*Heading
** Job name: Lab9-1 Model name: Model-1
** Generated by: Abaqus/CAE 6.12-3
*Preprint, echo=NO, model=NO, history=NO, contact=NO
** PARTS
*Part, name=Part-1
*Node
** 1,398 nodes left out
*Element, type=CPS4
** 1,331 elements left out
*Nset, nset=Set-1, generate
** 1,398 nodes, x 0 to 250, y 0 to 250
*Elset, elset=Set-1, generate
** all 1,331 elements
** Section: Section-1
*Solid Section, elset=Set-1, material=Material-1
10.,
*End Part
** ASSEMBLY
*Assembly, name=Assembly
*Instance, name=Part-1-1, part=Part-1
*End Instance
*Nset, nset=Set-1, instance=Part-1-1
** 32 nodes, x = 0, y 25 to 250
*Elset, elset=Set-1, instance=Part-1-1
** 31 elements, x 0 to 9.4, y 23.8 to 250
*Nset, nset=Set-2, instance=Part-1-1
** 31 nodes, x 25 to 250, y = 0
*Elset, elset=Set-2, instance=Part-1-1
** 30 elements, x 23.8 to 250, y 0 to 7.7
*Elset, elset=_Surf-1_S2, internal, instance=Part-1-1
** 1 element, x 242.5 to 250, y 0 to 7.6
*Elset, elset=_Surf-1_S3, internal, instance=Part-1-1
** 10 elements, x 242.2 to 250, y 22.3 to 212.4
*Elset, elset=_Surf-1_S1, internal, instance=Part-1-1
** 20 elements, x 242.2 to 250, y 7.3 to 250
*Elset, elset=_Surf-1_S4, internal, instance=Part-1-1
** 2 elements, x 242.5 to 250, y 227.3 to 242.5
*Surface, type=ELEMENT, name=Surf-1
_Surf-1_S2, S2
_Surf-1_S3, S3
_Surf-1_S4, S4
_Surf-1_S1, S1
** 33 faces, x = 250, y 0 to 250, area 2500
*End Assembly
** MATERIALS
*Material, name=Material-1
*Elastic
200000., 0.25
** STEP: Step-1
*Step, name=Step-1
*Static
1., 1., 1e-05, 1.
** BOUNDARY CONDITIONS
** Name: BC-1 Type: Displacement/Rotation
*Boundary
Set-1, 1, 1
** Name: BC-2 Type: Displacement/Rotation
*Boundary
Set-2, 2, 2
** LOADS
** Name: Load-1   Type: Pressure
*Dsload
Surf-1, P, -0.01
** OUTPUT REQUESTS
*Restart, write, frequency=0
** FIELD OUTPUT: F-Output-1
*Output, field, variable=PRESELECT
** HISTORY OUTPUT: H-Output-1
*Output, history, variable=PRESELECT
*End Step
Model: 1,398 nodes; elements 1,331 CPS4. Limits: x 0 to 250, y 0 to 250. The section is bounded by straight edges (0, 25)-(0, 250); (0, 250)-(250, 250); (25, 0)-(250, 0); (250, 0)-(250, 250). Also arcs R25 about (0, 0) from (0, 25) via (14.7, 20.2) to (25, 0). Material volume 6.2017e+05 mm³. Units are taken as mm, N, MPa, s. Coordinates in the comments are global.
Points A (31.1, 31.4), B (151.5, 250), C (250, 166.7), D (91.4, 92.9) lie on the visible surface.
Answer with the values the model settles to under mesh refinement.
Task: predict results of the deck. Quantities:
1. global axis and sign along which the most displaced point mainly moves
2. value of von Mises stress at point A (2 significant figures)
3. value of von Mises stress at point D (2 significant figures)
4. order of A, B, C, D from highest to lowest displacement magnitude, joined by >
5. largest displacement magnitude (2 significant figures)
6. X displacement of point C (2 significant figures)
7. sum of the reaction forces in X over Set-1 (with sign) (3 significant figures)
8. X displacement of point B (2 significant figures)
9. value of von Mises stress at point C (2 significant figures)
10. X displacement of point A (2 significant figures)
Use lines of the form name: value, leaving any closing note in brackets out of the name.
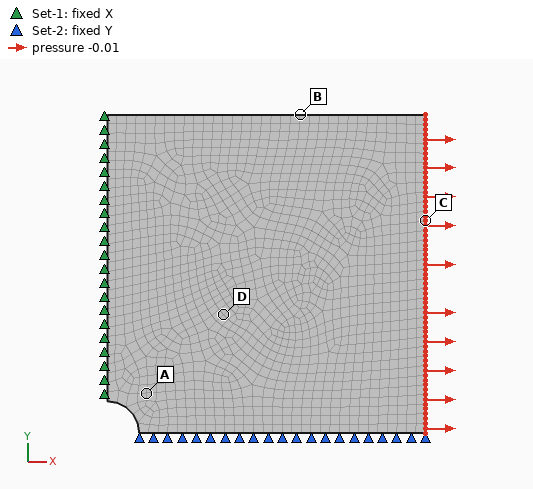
global axis and sign along which the most displaced point mainly moves: +X
value of von Mises stress at point A: 0.013 MPa
value of von Mises stress at point D: 0.011 MPa
order of A, B, C, D from highest to lowest displacement magnitude, joined by >: C > B > D > A
largest displacement magnitude: 1.3e-05 mm
X displacement of point C: 1.3e-05 mm
sum of the reaction forces in X over Set-1 (with sign): -25.0 N
X displacement of point B: 7.4e-06 mm
value of von Mises stress at point C: 0.010 MPa
X displacement of point A: 2.4e-06 mm
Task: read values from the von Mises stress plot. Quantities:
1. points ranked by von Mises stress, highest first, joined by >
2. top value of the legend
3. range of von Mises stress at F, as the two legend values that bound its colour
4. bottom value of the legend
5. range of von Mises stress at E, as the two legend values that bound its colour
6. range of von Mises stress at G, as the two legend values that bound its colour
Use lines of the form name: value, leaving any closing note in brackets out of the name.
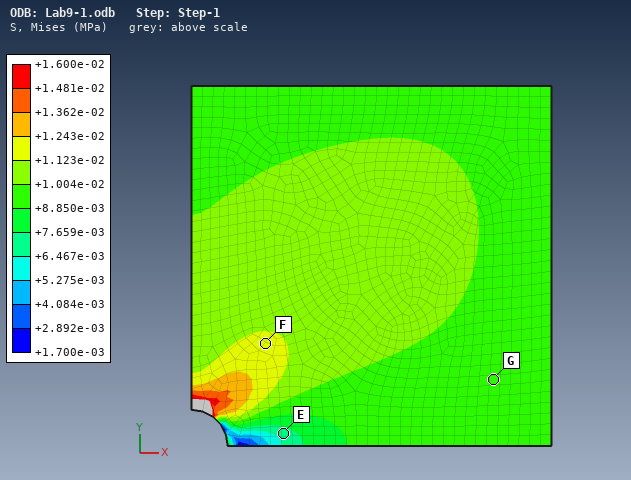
points ranked by von Mises stress, highest first, joined by >: F > G > E
top value of the legend: +1.600e-02 MPa
range of von Mises stress at F, as the two legend values that bound its colour: +1.123e-02 to +1.243e-02 MPa
bottom value of the legend: +1.700e-03 MPa
range of von Mises stress at E, as the two legend values that bound its colour: +6.467e-03 to +7.659e-03 MPa
range of von Mises stress at G, as the two legend values that bound its colour: +8.850e-03 to +1.004e-02 MPa
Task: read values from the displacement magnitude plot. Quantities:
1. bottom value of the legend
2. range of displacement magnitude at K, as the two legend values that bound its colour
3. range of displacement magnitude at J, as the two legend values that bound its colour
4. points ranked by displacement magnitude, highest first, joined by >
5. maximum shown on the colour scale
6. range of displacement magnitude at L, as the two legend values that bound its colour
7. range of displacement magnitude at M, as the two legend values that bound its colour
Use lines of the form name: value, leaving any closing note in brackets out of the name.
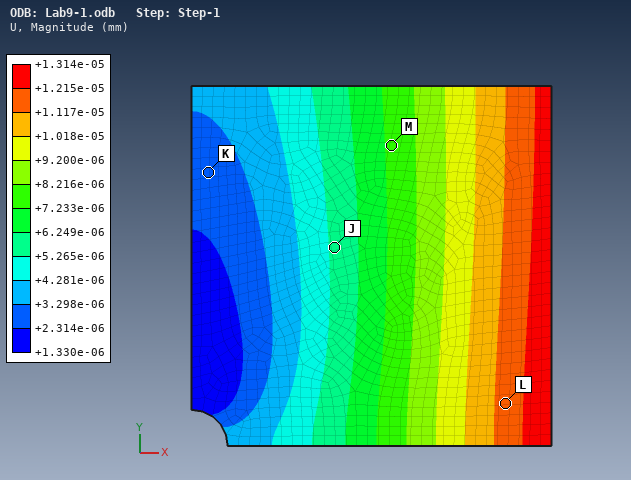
bottom value of the legend: +1.330e-06 mm
range of displacement magnitude at K, as the two legend values that bound its colour: +2.314e-06 to +3.298e-06 mm
range of displacement magnitude at J, as the two legend values that bound its colour: +5.265e-06 to +6.249e-06 mm
points ranked by displacement magnitude, highest first, joined by >: L > M > J > K
maximum shown on the colour scale: +1.314e-05 mm
range of displacement magnitude at L, as the two legend values that bound its colour: +1.117e-05 to +1.215e-05 mm
range of displacement magnitude at M, as the two legend values that bound its colour: +7.233e-06 to +8.216e-06 mm
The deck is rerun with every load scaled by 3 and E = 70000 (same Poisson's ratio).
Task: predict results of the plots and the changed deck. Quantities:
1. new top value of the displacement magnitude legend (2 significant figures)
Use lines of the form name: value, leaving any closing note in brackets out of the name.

new top value of the displacement magnitude legend: 1.1e-04 mm
